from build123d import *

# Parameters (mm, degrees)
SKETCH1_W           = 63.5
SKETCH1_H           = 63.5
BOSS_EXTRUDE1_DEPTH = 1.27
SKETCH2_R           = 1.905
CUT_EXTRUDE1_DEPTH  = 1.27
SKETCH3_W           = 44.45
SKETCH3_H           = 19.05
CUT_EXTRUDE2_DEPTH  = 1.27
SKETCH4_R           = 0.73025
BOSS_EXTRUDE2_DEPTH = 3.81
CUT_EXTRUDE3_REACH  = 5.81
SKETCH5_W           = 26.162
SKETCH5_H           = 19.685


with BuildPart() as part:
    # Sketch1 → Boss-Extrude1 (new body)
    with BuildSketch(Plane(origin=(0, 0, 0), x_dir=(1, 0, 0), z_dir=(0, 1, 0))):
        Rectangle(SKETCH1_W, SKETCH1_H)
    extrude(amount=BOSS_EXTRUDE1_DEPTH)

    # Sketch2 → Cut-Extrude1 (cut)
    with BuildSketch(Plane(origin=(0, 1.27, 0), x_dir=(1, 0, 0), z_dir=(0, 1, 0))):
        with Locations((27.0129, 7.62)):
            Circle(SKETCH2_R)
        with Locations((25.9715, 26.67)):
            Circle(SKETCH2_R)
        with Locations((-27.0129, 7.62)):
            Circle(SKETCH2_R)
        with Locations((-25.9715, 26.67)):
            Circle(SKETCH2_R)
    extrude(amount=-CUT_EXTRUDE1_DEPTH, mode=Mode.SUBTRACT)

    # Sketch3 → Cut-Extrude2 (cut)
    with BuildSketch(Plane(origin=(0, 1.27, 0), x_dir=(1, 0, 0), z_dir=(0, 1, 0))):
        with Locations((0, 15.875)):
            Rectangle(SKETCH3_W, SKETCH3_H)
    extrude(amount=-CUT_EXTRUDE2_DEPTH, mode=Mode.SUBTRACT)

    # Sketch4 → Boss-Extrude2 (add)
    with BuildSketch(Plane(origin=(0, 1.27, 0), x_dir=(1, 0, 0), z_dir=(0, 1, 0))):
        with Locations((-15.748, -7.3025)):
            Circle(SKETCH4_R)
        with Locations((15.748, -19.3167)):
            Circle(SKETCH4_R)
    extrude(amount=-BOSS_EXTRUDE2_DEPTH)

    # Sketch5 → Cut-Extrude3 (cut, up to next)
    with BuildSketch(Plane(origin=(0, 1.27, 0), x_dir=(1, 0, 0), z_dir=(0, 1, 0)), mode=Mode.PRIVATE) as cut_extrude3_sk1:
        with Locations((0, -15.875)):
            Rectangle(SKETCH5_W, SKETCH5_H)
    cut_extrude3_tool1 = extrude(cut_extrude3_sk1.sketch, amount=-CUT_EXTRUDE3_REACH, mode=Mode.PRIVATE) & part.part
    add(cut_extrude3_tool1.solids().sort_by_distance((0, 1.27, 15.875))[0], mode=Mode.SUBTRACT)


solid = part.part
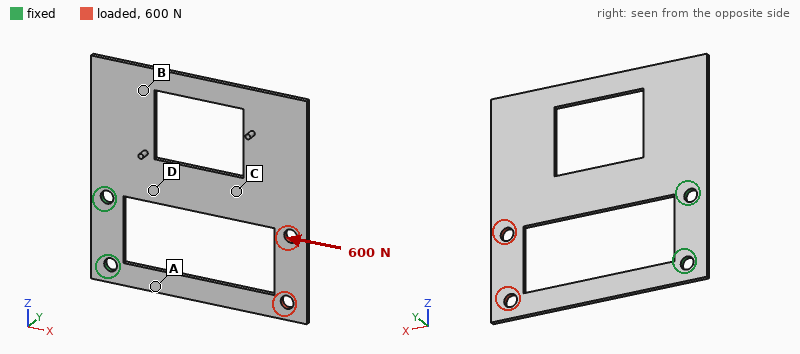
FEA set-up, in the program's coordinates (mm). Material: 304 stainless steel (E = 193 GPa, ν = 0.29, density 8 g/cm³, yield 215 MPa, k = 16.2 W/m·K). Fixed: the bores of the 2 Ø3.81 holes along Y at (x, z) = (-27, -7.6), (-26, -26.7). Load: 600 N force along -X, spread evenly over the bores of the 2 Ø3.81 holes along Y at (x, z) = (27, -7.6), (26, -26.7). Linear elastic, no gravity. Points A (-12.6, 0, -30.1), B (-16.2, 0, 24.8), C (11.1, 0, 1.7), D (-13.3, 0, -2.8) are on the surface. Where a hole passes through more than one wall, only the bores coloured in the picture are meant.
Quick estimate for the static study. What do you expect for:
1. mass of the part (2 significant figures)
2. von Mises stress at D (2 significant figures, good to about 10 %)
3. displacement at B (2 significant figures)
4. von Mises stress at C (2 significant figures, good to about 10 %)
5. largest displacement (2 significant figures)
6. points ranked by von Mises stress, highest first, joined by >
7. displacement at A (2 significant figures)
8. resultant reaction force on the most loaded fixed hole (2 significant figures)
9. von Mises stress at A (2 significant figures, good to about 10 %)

27 g
24 MPa
3.2 µm
17 MPa
14 µm
A > D > C > B
4.5 µm
310 N
38 MPa
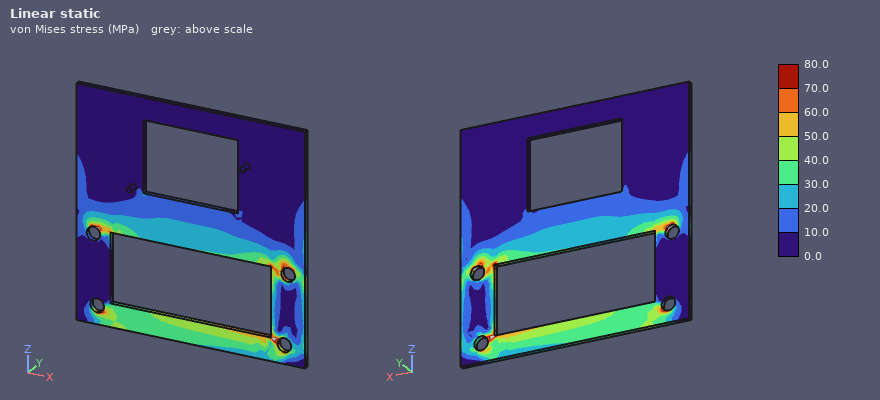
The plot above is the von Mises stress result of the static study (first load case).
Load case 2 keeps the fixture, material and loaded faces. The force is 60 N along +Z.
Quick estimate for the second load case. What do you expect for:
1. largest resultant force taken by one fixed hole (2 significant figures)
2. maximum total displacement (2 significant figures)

97 N
53 µm
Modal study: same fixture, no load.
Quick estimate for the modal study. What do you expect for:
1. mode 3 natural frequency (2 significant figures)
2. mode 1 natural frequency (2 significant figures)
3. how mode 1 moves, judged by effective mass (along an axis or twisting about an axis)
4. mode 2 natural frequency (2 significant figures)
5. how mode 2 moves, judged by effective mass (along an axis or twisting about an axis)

830 Hz
190 Hz
along Y
400 Hz
twisting about X
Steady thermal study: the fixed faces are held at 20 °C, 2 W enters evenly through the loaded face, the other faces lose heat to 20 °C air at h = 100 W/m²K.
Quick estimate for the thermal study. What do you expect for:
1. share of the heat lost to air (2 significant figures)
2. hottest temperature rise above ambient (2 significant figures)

100 %
31 K
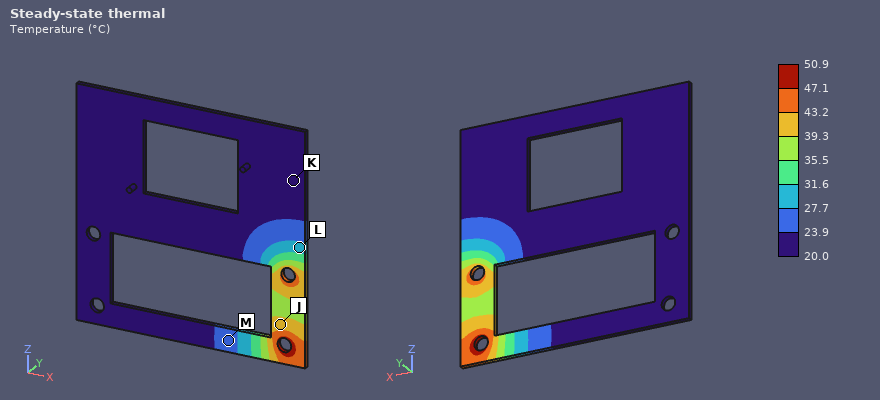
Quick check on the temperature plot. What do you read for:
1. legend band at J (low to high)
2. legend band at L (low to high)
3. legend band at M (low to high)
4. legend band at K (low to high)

39.3 to 43.2 °C
27.7 to 31.6 °C
23.9 to 27.7 °C
20.0 to 23.9 °C
